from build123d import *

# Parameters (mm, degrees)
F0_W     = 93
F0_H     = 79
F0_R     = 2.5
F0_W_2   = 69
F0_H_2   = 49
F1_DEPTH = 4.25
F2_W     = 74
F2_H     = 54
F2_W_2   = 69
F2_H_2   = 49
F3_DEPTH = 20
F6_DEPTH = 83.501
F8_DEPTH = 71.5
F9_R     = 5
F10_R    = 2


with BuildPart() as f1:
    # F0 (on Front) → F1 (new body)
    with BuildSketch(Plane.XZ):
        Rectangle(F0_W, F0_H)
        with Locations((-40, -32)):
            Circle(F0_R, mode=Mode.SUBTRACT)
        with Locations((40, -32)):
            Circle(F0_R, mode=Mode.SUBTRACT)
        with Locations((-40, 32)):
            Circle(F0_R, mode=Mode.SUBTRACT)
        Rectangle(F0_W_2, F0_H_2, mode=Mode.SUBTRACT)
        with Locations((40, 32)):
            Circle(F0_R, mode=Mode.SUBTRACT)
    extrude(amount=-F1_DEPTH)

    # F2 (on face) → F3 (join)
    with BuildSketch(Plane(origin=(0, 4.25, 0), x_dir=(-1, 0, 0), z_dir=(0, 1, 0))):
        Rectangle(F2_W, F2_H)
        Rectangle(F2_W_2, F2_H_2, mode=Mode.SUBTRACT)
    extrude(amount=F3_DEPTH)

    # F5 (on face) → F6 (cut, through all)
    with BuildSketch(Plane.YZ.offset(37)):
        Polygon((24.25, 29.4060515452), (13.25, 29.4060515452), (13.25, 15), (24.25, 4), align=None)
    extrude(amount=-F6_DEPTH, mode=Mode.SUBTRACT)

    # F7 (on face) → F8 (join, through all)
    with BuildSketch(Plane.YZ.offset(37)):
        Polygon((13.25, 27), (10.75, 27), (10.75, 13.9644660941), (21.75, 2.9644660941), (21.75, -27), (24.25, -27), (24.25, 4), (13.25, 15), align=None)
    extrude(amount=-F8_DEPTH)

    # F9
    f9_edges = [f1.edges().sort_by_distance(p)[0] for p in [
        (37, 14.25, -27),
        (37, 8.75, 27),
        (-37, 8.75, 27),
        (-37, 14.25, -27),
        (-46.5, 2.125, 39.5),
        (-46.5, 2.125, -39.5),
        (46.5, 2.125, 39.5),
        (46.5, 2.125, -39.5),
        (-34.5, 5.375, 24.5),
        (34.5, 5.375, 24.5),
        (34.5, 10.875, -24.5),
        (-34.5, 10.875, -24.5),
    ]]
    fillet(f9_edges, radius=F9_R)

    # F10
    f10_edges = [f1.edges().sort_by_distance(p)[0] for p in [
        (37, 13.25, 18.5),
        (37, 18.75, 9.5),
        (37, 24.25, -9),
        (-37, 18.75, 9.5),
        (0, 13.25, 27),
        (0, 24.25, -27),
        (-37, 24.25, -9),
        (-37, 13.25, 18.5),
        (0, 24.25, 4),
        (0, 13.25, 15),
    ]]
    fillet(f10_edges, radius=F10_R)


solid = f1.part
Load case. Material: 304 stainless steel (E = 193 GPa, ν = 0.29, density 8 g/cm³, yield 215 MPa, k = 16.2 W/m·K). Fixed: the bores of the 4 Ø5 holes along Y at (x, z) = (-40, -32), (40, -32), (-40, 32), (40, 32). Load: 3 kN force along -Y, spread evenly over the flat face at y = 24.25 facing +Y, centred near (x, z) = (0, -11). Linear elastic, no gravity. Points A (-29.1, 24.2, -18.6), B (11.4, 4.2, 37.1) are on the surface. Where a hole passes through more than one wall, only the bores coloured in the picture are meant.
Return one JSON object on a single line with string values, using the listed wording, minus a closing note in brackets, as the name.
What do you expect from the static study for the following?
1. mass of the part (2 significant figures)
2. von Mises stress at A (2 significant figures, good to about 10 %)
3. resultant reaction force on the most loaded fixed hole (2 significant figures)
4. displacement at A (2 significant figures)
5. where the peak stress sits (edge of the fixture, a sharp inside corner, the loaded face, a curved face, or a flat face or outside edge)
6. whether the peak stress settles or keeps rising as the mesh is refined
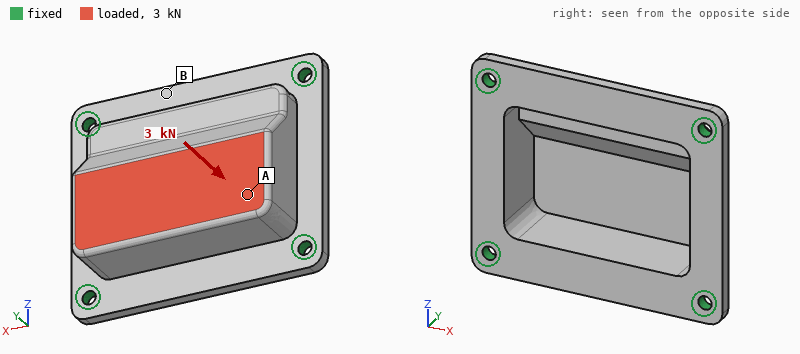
{"mass of the part": "280 g", "von Mises stress at A": "23 MPa", "resultant reaction force on the most loaded fixed hole": "1.2 kN", "displacement at A": "13 µm", "where the peak stress sits": "edge of the fixture", "whether the peak stress settles or keeps rising as the mesh is refined": "keeps rising"}
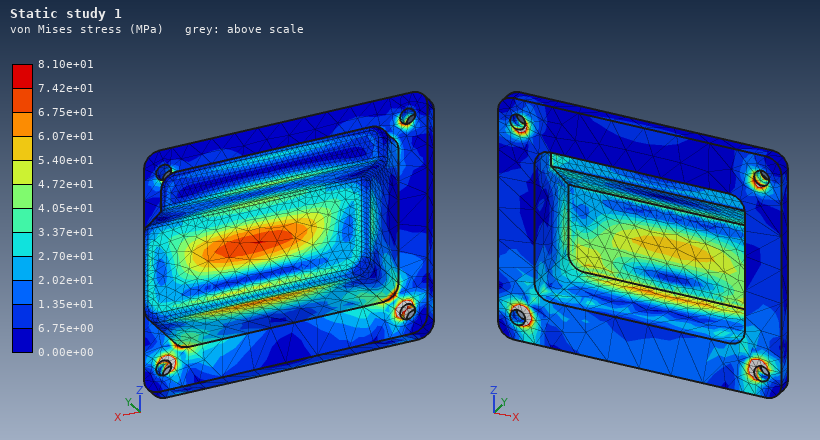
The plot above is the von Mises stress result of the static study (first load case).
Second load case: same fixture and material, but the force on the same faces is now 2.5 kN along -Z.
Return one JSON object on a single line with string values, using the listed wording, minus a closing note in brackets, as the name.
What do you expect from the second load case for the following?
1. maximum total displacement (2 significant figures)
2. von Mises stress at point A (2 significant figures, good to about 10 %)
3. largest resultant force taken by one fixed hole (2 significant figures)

{"maximum total displacement": "16 µm", "von Mises stress at point A": "12 MPa", "largest resultant force taken by one fixed hole": "890 N"}
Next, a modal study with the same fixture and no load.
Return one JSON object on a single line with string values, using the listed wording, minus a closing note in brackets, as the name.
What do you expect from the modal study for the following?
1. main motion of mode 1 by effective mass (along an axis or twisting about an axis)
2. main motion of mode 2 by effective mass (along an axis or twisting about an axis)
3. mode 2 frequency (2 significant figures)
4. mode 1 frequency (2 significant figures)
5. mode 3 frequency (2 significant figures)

{"main motion of mode 1 by effective mass": "along Y", "main motion of mode 2 by effective mass": "along Y", "mode 2 frequency": "6200 Hz", "mode 1 frequency": "4800 Hz", "mode 3 frequency": "6800 Hz"}
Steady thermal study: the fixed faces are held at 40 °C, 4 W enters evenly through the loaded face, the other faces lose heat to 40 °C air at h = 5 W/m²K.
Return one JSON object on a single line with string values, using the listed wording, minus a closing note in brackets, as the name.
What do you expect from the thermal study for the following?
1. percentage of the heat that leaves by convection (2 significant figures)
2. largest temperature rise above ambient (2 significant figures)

{"percentage of the heat that leaves by convection": "26 %", "largest temperature rise above ambient": "23 K"}
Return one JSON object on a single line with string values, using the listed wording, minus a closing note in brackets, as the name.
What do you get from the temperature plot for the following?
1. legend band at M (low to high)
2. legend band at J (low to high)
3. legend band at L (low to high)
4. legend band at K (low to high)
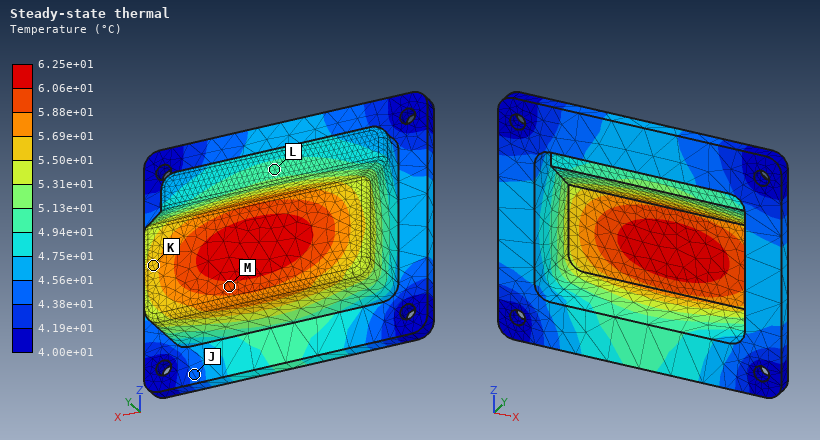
{"legend band at M": "5.88e+01 to 6.06e+01 °C", "legend band at J": "4.38e+01 to 4.56e+01 °C", "legend band at L": "4.94e+01 to 5.13e+01 °C", "legend band at K": "5.50e+01 to 5.69e+01 °C"}
